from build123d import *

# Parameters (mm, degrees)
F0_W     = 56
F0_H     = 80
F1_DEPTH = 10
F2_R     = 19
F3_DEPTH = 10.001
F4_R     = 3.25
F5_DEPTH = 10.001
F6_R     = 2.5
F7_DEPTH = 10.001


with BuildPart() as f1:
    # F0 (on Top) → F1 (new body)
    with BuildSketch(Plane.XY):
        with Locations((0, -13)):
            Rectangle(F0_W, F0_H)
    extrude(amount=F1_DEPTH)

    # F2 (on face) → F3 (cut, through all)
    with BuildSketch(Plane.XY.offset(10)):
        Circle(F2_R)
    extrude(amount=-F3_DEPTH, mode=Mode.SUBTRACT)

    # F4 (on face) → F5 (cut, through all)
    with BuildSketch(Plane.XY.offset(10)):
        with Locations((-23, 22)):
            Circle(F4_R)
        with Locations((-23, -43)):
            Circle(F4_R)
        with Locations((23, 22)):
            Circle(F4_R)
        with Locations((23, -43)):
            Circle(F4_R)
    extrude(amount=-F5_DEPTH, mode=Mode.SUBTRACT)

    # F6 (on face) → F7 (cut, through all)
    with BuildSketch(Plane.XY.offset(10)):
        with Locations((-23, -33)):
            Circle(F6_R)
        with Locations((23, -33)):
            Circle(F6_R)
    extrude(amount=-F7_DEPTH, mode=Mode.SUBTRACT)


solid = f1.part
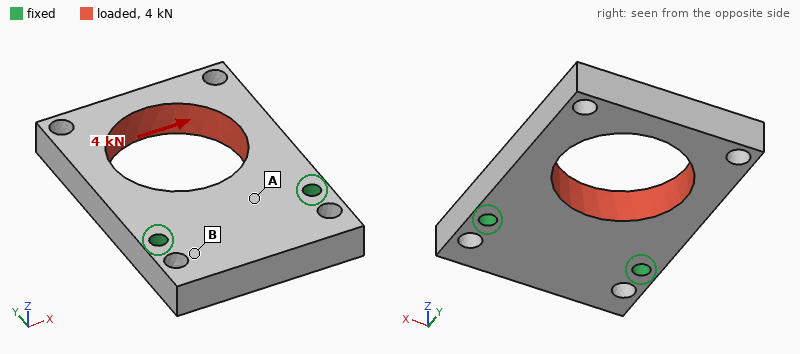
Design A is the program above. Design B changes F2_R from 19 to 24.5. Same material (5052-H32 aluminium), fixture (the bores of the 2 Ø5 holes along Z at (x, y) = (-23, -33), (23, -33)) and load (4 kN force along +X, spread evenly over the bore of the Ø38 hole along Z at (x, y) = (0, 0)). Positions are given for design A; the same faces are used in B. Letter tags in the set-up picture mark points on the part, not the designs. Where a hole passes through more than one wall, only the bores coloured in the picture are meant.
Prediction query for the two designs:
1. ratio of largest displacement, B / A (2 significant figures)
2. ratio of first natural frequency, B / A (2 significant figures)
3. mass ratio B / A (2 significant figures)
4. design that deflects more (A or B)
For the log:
5.9
0.94
0.76
B
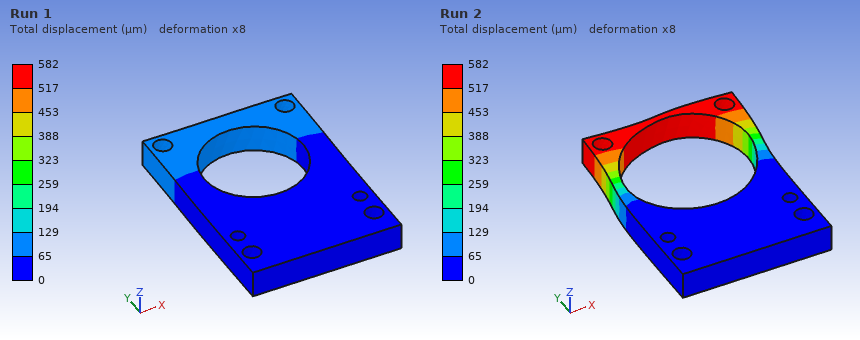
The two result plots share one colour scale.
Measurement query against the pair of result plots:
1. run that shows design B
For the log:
Run 2
